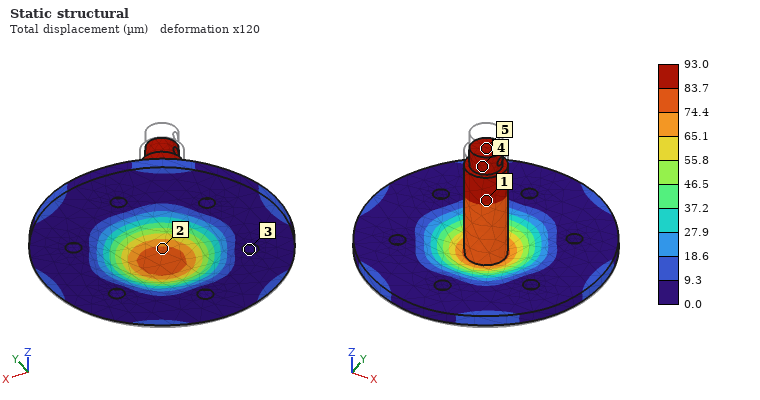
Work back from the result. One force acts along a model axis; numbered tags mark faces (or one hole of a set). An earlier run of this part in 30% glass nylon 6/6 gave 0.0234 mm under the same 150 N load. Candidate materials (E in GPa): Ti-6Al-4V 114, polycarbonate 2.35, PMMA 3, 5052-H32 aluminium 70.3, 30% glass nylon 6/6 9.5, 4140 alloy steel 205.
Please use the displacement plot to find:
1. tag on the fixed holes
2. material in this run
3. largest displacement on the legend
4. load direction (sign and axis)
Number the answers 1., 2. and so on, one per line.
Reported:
1. 3
2. polycarbonate
3. 93.0 µm
4. -Z
